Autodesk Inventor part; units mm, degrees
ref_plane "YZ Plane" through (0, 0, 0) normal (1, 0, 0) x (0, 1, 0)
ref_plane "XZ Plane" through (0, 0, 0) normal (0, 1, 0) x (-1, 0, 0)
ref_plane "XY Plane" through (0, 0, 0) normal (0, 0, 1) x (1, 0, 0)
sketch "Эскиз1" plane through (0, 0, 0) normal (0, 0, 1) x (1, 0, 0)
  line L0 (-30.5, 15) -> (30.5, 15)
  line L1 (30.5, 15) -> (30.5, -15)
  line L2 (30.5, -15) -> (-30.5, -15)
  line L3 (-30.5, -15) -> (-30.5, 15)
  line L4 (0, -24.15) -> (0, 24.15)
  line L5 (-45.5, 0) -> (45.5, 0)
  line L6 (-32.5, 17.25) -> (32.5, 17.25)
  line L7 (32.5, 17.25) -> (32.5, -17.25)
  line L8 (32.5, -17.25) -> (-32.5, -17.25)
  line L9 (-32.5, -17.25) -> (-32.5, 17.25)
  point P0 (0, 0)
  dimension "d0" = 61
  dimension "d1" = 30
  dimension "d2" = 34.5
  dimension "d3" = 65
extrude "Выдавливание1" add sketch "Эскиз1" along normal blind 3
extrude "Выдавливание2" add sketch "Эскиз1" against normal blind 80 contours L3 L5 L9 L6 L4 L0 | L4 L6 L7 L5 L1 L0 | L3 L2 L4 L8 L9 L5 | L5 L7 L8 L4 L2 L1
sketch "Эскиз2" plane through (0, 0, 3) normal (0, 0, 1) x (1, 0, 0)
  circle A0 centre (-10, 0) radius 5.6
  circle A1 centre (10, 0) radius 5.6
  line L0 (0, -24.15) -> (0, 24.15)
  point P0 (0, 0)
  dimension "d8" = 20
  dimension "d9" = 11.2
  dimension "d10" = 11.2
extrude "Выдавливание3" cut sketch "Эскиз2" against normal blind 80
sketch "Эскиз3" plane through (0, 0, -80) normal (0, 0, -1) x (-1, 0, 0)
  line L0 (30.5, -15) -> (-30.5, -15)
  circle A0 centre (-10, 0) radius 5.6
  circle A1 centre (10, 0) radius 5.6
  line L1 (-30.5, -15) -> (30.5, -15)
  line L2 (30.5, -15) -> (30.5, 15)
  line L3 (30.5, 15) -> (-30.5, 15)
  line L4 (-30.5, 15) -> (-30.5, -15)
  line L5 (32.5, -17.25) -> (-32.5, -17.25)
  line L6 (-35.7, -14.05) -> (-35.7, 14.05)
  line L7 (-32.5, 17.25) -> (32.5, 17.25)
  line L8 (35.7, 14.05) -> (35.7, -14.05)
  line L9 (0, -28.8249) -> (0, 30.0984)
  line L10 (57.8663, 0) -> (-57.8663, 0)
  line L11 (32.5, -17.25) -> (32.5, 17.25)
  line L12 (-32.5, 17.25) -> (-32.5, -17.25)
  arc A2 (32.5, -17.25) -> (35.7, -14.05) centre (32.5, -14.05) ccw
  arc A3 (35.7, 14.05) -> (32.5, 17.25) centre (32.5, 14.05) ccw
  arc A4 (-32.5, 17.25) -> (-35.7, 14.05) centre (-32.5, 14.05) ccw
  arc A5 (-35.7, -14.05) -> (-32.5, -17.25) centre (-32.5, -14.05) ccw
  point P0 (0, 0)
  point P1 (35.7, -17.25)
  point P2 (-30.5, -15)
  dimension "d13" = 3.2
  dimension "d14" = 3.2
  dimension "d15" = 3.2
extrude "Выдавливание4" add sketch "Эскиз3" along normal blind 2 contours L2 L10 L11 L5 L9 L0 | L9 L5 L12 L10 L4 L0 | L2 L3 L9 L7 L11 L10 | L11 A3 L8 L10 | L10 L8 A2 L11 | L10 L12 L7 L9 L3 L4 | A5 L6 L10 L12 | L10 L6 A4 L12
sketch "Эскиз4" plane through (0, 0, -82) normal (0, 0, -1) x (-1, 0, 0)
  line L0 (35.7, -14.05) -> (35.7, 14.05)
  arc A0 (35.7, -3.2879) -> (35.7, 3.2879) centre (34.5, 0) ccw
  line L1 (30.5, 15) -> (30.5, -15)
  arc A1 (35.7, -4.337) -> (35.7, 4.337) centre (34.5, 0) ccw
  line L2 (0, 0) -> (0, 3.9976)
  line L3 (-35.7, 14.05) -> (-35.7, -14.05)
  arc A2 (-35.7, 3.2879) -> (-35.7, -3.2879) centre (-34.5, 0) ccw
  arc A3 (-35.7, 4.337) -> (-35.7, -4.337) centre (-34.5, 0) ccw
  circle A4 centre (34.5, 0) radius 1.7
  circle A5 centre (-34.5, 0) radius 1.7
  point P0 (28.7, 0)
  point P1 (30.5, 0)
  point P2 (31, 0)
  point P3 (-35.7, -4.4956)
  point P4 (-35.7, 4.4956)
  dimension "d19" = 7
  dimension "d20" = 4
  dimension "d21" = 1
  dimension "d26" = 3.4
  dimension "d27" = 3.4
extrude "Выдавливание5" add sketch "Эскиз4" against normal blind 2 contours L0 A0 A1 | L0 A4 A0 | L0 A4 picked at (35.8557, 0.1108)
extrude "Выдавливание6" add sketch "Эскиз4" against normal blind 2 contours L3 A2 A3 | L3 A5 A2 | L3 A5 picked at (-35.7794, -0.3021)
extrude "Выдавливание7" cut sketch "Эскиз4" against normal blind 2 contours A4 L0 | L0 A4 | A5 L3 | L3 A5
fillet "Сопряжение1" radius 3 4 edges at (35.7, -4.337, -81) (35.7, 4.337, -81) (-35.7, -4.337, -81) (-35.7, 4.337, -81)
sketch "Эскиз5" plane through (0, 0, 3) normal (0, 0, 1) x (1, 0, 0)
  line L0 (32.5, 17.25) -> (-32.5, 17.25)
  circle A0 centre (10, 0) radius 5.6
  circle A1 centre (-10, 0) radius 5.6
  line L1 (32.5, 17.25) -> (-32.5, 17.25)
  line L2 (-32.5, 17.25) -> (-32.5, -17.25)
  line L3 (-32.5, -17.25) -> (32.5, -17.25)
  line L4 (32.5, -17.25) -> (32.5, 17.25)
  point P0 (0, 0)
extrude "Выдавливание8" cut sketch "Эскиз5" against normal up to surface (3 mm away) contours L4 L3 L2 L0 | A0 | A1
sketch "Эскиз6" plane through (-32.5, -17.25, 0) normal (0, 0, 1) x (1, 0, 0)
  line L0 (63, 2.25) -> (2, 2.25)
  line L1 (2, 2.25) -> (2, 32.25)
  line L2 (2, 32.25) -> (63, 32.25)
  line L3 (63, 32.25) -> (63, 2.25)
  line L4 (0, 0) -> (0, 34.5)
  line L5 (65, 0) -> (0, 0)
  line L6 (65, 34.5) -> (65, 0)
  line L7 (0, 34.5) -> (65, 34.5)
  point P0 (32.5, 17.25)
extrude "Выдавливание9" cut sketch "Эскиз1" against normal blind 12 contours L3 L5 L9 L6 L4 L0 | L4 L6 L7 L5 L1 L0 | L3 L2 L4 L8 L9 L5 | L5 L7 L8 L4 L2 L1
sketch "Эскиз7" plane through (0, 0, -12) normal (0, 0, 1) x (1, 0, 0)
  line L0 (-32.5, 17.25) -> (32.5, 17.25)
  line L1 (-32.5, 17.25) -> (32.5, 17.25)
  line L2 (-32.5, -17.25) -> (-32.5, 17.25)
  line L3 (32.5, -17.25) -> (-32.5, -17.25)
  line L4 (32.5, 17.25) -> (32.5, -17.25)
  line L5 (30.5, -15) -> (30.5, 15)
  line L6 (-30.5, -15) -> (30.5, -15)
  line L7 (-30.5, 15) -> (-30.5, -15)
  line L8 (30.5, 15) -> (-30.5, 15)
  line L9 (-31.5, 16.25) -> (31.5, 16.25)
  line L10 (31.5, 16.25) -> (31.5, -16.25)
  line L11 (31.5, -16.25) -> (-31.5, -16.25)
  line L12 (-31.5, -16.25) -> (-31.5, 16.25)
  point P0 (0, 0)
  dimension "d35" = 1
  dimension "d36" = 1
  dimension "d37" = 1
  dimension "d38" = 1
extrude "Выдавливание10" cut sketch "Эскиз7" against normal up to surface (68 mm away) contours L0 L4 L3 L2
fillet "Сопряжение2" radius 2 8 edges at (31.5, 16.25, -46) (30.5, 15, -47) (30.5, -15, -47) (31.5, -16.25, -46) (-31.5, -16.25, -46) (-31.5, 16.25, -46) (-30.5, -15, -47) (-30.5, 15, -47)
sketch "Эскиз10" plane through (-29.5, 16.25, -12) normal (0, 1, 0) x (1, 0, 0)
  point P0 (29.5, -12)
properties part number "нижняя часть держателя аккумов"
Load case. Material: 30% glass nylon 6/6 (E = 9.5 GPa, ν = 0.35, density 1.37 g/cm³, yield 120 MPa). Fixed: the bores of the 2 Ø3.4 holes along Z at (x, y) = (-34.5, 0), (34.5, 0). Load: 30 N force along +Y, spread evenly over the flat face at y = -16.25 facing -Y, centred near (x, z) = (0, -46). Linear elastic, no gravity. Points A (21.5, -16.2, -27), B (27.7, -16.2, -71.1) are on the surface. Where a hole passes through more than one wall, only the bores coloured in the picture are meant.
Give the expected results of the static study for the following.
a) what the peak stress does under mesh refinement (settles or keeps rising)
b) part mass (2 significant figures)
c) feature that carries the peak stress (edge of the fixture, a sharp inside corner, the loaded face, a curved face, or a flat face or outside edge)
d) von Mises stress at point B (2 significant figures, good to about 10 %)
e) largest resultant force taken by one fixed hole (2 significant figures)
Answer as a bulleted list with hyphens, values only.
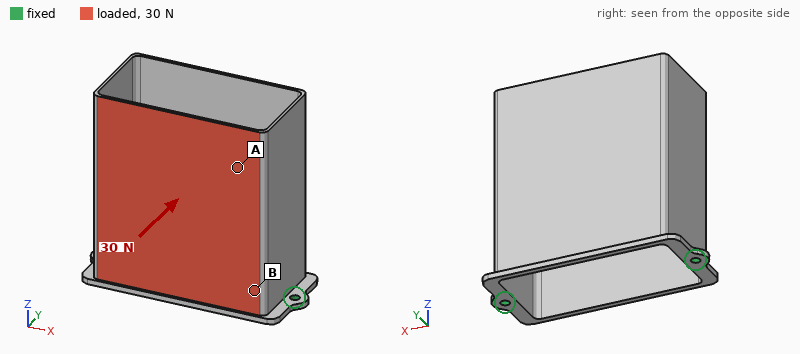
- keeps rising
- 22 g
- edge of the fixture
- 4.1 MPa
- 16 N
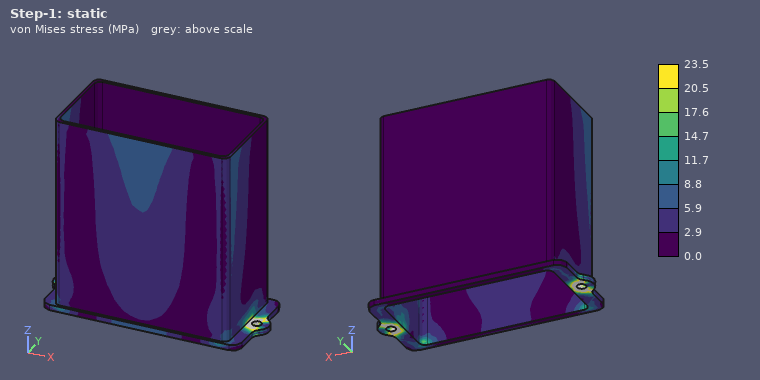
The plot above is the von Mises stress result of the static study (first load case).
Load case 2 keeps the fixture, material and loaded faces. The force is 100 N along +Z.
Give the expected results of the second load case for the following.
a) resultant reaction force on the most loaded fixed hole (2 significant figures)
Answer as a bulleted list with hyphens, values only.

- 50 N
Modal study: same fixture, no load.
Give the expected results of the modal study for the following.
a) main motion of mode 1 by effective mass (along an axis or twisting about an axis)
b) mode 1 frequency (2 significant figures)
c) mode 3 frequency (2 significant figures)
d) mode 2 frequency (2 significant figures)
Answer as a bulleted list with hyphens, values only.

- along Y
- 260 Hz
- 580 Hz
- 530 Hz
